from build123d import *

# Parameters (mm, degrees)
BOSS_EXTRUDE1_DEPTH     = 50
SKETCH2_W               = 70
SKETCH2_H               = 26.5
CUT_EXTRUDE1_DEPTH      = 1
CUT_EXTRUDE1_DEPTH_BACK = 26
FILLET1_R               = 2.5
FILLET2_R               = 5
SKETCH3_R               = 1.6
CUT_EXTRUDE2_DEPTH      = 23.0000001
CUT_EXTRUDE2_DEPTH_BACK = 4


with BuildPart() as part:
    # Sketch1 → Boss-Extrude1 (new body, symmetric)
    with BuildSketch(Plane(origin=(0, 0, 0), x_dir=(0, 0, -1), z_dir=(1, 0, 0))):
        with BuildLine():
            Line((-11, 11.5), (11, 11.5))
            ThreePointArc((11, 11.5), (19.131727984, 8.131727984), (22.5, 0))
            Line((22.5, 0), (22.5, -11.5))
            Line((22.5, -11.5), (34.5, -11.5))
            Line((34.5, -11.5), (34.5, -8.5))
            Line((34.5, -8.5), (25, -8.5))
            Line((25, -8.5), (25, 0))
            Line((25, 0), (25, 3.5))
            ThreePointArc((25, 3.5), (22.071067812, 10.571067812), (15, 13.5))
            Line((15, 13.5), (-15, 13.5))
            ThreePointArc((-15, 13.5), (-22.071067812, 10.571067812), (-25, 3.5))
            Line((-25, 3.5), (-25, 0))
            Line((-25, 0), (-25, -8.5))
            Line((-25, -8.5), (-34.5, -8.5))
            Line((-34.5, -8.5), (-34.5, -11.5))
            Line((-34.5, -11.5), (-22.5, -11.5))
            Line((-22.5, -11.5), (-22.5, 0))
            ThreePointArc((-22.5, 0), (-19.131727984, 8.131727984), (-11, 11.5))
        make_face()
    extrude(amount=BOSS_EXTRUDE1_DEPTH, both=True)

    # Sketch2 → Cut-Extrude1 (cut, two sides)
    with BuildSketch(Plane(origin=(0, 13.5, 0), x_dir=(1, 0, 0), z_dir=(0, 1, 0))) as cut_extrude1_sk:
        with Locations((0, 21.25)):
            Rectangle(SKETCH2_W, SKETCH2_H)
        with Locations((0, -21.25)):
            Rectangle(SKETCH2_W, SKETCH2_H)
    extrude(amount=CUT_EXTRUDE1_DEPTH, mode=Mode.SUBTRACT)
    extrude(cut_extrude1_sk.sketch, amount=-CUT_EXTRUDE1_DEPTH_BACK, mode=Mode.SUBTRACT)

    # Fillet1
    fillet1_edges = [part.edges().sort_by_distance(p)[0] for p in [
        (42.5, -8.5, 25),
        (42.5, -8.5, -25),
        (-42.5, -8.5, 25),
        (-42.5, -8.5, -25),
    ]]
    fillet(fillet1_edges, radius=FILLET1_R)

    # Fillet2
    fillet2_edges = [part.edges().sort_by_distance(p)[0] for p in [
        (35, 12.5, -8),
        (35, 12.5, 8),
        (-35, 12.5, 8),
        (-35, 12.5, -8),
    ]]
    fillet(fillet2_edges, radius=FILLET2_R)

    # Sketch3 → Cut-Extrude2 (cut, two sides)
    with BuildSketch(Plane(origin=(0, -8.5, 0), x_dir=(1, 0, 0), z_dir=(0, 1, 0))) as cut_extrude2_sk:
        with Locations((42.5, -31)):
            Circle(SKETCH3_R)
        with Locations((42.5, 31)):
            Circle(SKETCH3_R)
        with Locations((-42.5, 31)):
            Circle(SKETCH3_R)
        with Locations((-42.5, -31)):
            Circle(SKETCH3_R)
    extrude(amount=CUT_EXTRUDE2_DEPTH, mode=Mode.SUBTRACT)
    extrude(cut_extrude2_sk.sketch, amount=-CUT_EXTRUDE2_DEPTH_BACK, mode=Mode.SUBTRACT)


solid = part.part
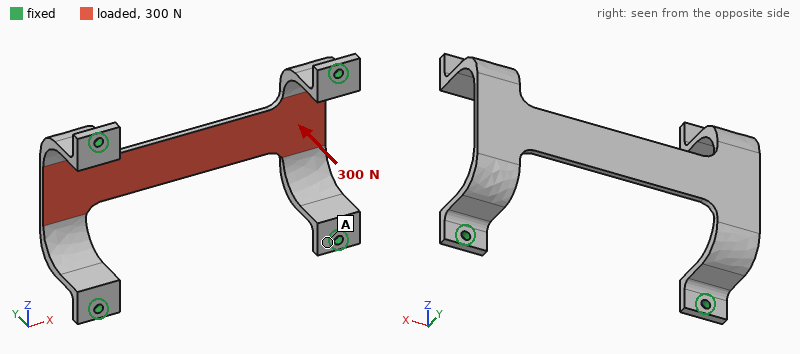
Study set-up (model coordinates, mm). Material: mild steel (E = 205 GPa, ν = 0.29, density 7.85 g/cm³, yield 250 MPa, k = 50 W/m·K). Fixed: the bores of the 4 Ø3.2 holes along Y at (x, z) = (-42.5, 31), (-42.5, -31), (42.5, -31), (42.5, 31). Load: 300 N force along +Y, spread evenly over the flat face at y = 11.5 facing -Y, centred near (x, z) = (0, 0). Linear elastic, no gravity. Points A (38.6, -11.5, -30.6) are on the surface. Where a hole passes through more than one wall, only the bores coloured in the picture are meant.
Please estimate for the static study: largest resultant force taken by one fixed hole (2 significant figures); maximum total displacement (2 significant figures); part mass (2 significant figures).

110 N
0.15 mm
85 g
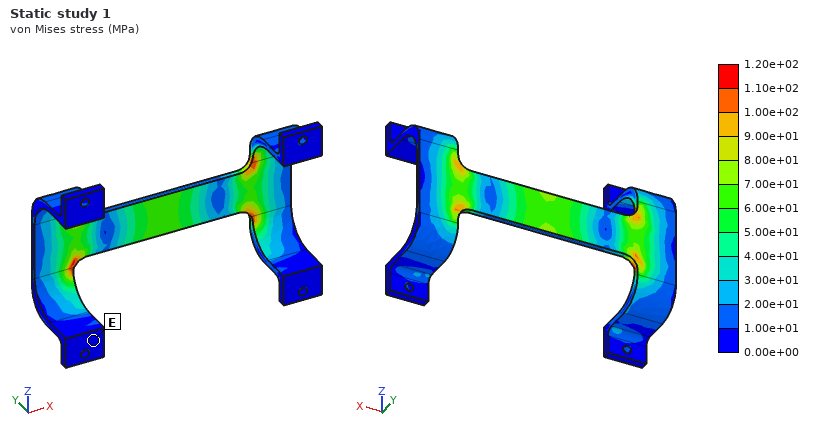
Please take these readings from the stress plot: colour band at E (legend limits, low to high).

0.00e+00 to 1.00e+01 MPa
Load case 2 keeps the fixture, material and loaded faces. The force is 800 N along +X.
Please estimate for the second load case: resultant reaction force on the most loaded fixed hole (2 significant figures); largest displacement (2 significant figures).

200 N
64 µm
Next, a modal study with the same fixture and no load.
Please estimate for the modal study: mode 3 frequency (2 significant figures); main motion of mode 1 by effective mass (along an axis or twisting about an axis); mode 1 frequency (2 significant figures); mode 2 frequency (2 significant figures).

2500 Hz
along Y
1500 Hz
2500 Hz
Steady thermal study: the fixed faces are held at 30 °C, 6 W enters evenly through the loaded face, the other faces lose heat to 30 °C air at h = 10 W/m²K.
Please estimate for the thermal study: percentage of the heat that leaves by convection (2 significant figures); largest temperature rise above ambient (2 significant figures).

21 %
44 K
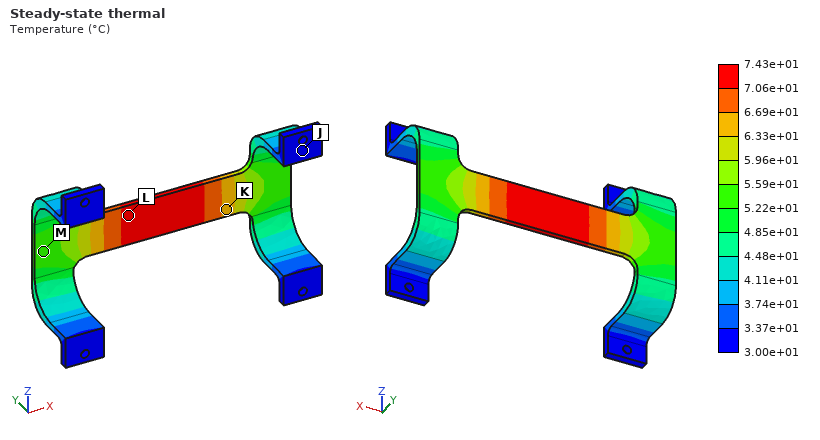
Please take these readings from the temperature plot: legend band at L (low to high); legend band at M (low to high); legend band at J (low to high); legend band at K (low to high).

7.06e+01 to 7.43e+01 °C
5.22e+01 to 5.59e+01 °C
3.00e+01 to 3.37e+01 °C
6.33e+01 to 6.69e+01 °C
